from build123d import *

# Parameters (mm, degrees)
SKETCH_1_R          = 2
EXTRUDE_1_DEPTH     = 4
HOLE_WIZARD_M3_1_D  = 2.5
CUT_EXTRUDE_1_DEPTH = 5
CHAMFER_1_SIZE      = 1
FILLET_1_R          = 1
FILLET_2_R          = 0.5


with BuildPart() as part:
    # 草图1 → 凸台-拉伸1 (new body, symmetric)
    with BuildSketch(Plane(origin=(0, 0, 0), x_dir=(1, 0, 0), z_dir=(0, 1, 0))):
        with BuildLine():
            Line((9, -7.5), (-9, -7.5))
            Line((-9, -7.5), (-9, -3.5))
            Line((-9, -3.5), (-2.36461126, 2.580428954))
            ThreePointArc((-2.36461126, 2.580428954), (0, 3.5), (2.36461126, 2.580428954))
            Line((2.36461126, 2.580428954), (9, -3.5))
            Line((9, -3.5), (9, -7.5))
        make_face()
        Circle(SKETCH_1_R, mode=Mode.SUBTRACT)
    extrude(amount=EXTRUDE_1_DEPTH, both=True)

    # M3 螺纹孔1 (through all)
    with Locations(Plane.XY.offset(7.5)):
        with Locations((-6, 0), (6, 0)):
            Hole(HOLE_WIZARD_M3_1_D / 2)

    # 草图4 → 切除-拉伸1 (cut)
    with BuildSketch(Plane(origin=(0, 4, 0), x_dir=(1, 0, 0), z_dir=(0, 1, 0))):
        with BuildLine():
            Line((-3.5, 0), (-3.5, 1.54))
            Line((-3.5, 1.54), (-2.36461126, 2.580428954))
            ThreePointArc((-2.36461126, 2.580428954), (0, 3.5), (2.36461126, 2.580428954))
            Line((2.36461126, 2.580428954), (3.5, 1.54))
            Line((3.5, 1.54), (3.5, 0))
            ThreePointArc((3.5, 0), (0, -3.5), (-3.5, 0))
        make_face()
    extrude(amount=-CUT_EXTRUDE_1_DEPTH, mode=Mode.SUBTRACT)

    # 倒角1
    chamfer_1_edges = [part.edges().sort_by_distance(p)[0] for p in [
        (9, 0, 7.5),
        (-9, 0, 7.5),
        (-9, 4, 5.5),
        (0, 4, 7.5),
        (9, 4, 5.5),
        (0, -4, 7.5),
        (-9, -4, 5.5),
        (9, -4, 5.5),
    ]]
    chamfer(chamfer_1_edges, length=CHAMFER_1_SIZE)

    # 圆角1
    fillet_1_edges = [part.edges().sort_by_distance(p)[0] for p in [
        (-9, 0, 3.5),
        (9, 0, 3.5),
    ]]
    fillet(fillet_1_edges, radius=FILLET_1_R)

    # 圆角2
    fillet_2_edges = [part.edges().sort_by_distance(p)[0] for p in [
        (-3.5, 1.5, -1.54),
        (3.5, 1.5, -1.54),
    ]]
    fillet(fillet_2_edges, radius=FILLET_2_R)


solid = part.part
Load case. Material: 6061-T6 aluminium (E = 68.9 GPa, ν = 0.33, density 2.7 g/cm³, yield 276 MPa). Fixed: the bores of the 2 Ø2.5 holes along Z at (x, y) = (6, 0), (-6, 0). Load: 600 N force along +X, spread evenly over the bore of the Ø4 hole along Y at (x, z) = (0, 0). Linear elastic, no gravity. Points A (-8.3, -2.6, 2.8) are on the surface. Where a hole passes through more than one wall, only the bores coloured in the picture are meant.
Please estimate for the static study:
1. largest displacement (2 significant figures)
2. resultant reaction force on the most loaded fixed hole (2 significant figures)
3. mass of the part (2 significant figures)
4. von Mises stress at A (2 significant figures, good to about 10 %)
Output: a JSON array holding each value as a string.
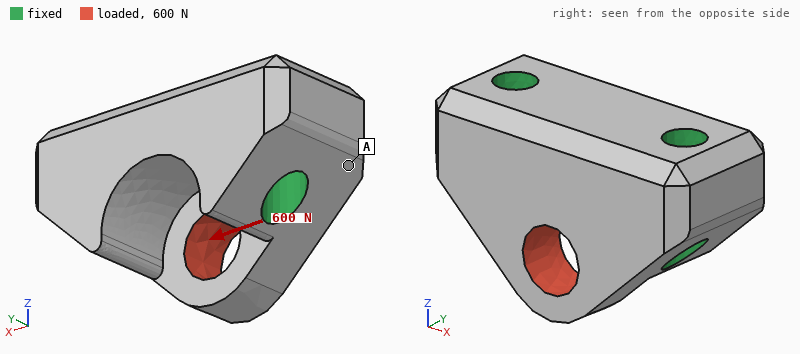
["5.6 µm", "330 N", "2.2 g", "8.2 MPa"]
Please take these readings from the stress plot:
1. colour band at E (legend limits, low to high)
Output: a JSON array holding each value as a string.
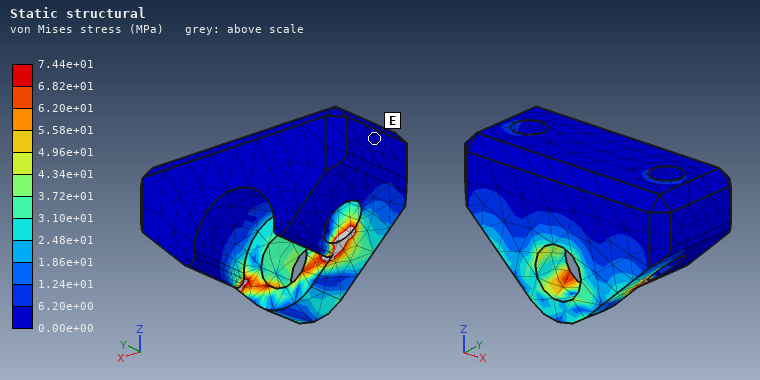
["0.00e+00 to 6.20e+00 MPa"]
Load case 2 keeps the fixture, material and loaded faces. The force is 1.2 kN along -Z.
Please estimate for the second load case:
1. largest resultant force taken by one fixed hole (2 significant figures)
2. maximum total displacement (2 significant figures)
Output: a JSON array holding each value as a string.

["610 N", "9.7 µm"]
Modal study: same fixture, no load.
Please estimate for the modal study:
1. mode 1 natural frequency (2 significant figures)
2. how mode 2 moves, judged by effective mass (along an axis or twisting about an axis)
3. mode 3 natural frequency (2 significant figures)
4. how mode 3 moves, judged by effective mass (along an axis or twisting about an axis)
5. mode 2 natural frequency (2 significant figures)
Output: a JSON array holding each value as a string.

["79 kHz", "along Y", "120 kHz", "along Z", "110 kHz"]
